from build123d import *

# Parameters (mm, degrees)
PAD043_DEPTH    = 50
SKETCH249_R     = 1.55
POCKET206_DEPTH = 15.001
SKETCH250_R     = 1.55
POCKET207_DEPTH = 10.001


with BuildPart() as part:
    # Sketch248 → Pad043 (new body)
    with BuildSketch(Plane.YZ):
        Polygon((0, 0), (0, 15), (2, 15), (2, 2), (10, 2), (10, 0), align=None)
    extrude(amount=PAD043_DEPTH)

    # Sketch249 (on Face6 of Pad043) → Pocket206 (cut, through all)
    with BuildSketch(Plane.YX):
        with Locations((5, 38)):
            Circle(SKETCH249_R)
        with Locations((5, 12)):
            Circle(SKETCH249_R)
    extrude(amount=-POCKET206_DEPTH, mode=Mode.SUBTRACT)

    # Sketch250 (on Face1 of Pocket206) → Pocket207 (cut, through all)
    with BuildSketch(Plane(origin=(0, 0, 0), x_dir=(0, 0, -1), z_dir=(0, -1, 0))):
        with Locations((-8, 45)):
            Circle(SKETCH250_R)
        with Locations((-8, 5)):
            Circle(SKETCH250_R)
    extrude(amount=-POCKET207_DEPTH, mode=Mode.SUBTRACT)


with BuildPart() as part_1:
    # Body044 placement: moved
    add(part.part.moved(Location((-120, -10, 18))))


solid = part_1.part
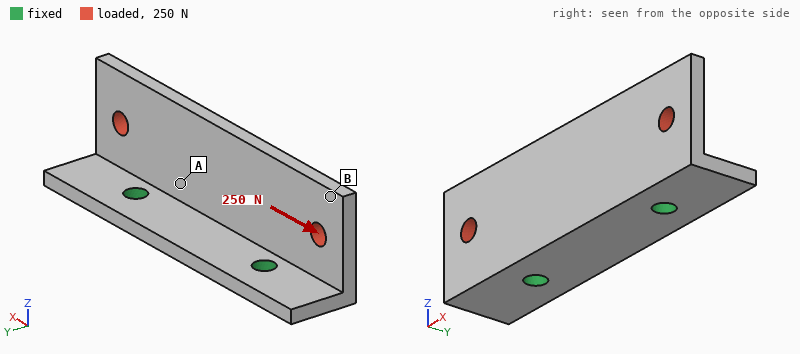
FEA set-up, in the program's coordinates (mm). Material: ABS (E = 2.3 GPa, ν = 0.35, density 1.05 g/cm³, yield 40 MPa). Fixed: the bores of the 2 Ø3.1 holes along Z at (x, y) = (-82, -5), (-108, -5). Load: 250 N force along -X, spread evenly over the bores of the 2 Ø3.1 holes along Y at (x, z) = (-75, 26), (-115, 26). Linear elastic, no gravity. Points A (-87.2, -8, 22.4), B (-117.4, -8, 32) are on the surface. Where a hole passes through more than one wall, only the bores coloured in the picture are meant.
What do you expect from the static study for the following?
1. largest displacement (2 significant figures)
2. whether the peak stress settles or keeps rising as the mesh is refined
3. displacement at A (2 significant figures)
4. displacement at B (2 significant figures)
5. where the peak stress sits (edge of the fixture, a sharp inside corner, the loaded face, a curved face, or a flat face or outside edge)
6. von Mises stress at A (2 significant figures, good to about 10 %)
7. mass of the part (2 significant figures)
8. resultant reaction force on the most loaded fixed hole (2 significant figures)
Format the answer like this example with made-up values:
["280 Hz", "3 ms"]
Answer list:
["0.25 mm", "keeps rising", "0.056 mm", "0.22 mm", "edge of the fixture", "8.1 MPa", "2.4 g", "140 N"]
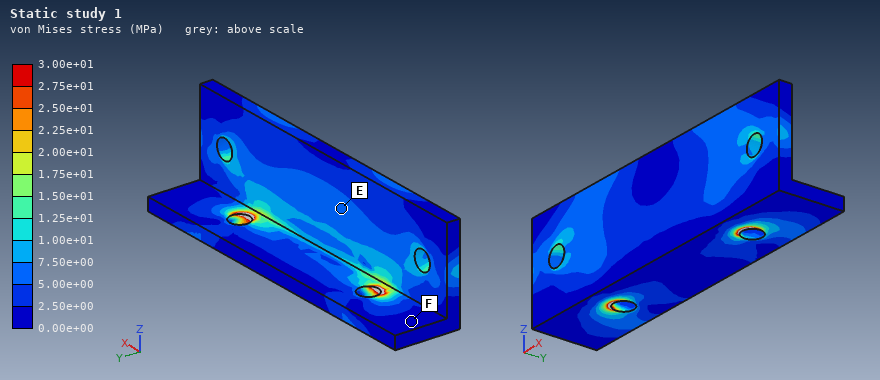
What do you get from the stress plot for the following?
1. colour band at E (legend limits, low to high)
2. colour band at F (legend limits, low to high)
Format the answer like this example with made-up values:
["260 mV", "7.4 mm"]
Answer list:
["5.00e+00 to 7.50e+00 MPa", "0.00e+00 to 2.50e+00 MPa"]
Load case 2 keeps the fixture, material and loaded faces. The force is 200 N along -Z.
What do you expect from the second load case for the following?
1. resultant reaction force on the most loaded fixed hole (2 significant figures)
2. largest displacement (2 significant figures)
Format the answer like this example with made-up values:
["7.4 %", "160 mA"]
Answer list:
["110 N", "0.46 mm"]
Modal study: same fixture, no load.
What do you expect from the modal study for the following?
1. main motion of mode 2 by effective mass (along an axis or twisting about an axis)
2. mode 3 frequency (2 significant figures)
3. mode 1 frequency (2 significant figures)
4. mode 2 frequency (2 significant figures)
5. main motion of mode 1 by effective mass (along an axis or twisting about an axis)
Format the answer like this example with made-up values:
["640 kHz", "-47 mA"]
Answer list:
["twisting about Z", "3200 Hz", "1600 Hz", "2100 Hz", "along Y"]
